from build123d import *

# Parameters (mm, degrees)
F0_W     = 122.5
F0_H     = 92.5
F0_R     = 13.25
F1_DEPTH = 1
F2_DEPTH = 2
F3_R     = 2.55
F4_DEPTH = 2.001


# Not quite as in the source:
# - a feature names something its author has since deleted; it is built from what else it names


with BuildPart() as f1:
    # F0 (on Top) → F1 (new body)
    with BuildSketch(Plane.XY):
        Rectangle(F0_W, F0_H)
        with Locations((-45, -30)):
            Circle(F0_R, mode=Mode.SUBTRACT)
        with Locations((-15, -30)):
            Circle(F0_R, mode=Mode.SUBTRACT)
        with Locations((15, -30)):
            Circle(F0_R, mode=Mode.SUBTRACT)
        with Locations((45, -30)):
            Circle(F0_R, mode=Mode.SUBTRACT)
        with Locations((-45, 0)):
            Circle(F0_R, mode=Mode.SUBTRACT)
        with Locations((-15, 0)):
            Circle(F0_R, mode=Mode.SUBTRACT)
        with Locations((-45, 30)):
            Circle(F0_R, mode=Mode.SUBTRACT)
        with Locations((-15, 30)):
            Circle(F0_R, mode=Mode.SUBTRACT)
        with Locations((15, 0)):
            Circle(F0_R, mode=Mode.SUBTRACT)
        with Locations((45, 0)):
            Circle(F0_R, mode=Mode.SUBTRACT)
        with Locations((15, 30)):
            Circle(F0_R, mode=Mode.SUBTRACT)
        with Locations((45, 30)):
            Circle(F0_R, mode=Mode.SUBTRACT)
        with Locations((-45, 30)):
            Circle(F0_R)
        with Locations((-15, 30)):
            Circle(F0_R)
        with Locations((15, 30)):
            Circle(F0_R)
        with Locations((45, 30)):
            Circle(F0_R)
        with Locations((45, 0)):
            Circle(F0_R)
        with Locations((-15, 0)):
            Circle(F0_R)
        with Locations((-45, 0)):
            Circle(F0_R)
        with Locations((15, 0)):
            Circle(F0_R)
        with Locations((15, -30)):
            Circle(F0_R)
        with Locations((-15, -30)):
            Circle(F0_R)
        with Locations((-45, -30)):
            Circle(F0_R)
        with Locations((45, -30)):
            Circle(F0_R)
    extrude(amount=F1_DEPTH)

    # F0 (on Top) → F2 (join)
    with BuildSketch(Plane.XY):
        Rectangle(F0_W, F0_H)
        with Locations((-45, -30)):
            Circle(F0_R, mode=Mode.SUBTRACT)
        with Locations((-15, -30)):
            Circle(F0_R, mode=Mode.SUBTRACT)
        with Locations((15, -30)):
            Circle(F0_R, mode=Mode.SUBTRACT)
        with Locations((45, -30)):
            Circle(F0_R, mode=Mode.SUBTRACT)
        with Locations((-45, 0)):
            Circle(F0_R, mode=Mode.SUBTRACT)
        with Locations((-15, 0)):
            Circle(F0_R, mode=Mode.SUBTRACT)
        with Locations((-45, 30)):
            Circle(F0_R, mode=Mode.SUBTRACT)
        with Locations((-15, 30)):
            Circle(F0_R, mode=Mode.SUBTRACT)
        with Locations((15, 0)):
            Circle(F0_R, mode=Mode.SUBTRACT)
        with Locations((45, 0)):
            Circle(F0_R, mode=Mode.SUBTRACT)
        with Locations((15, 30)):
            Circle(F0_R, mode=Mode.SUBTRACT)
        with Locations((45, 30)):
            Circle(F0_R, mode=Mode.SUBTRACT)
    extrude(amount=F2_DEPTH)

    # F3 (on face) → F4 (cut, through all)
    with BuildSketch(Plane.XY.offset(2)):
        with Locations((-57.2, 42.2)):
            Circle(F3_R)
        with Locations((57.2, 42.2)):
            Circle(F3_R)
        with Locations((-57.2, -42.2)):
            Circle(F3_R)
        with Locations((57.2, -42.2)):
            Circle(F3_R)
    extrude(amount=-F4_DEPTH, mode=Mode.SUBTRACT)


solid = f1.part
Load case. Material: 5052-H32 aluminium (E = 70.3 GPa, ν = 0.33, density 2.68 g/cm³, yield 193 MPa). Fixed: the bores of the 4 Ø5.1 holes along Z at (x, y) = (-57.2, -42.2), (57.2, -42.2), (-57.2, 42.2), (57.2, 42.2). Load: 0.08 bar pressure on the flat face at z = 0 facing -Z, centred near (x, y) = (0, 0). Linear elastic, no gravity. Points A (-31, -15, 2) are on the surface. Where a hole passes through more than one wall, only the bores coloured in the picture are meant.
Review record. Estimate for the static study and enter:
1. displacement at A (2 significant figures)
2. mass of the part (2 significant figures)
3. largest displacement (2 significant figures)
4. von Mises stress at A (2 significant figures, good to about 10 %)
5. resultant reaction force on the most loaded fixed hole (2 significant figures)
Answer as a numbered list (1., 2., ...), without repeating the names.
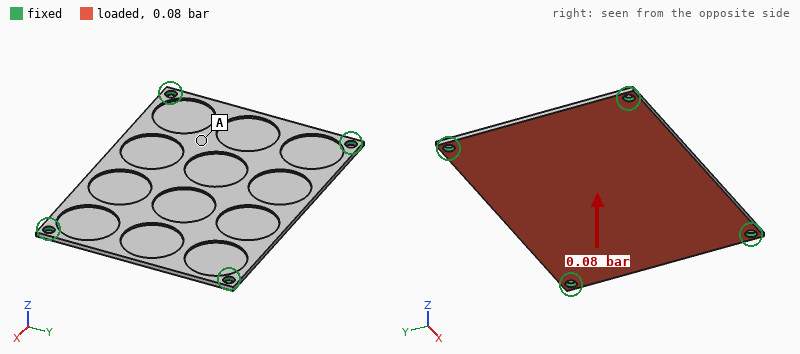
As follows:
1. 0.20 mm
2. 43 g
3. 0.32 mm
4. 6.3 MPa
5. 25 N
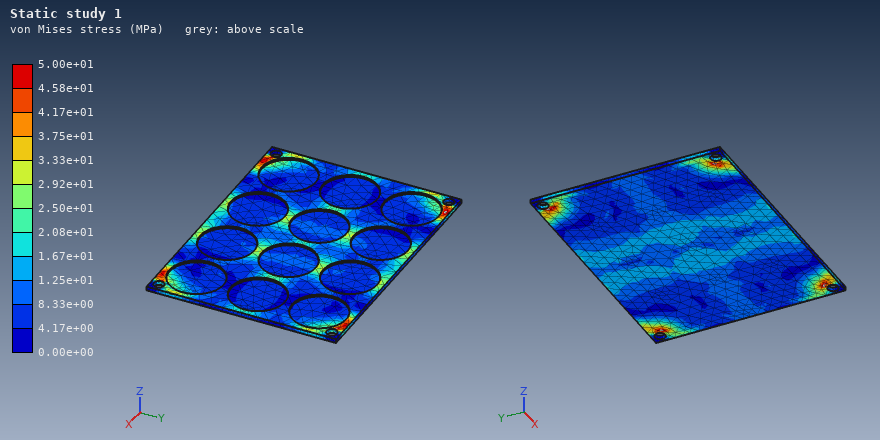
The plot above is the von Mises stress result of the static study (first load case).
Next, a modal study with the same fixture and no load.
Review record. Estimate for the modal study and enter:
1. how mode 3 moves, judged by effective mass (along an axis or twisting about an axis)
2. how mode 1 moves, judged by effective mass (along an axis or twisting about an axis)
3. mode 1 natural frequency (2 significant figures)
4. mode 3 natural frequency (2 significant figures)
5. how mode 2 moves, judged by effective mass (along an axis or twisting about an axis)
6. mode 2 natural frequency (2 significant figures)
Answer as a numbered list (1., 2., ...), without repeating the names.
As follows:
1. twisting about Y
2. along Z
3. 490 Hz
4. 1100 Hz
5. twisting about X
6. 840 Hz
